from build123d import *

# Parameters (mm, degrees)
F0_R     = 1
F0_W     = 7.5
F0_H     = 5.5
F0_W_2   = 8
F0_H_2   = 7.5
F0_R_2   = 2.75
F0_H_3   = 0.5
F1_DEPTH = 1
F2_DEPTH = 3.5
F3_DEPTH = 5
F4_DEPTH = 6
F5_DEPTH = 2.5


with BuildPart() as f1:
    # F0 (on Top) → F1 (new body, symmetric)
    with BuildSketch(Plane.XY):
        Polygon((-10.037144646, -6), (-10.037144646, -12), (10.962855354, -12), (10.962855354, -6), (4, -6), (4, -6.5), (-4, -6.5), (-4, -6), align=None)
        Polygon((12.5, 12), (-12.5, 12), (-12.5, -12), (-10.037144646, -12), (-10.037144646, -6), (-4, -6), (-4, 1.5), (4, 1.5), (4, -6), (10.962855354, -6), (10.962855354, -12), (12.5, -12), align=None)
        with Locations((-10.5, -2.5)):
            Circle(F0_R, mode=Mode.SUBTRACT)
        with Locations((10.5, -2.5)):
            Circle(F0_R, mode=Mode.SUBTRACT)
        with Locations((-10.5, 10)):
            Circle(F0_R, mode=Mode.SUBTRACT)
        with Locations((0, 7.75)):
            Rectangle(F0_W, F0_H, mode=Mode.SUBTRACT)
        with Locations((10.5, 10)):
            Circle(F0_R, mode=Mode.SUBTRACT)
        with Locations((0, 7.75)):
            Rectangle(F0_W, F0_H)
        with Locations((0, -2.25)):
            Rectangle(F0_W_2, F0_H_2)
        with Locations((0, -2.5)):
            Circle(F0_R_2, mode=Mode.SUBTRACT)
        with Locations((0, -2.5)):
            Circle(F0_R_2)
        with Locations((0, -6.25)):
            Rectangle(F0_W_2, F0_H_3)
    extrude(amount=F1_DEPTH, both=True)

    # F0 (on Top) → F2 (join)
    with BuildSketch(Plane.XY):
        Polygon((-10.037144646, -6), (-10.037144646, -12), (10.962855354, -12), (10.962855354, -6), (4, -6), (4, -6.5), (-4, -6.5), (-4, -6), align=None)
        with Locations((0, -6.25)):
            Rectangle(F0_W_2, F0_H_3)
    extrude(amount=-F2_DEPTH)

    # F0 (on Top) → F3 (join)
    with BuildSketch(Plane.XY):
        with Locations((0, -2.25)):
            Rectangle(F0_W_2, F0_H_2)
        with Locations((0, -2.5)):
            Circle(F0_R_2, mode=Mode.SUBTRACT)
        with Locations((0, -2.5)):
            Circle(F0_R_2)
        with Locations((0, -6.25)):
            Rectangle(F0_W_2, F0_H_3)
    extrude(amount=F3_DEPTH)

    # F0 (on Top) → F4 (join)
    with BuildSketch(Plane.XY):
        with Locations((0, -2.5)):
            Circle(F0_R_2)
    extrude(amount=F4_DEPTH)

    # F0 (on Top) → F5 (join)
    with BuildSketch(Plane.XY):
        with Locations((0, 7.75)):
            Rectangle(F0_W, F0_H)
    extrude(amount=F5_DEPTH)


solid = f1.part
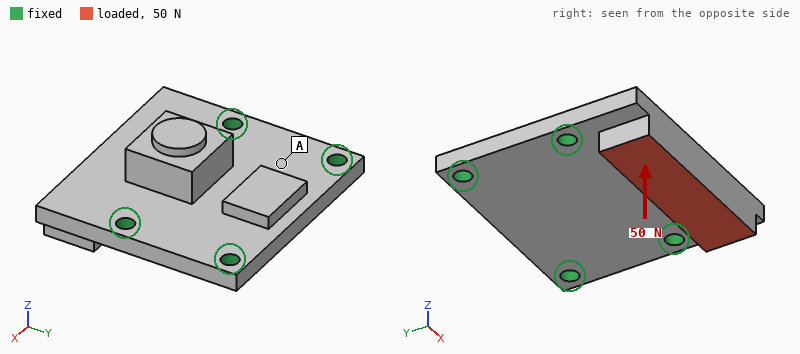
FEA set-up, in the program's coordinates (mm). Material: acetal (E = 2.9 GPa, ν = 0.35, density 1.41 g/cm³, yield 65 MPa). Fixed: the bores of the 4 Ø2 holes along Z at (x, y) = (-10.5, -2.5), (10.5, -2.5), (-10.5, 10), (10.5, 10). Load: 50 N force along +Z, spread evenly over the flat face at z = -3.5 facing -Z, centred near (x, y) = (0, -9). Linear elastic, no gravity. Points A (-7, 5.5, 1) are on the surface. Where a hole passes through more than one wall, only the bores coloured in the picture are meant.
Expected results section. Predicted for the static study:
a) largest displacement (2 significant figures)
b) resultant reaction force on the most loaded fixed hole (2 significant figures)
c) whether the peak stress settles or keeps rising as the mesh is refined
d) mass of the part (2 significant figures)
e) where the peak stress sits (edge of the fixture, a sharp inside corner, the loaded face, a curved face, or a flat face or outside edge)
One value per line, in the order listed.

0.19 mm
32 N
keeps rising
2.6 g
edge of the fixture
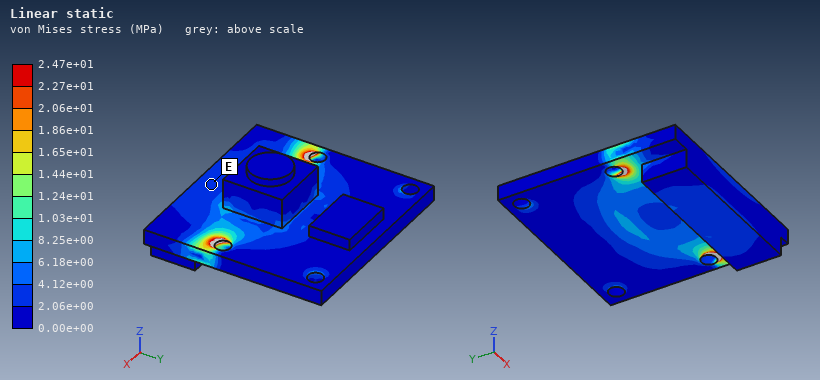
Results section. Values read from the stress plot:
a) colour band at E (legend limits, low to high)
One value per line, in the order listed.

2.06e+00 to 4.12e+00 MPa
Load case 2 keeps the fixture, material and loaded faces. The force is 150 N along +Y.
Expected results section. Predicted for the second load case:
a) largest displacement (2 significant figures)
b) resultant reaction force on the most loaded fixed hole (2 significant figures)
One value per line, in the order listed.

0.36 mm
63 N
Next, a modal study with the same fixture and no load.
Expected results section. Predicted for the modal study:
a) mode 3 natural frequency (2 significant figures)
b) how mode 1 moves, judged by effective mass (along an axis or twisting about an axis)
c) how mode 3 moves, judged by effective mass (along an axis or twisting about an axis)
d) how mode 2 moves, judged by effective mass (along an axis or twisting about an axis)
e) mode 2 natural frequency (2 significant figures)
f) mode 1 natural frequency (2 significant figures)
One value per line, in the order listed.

7700 Hz
along Z
twisting about Y
along Z
6000 Hz
3200 Hz
